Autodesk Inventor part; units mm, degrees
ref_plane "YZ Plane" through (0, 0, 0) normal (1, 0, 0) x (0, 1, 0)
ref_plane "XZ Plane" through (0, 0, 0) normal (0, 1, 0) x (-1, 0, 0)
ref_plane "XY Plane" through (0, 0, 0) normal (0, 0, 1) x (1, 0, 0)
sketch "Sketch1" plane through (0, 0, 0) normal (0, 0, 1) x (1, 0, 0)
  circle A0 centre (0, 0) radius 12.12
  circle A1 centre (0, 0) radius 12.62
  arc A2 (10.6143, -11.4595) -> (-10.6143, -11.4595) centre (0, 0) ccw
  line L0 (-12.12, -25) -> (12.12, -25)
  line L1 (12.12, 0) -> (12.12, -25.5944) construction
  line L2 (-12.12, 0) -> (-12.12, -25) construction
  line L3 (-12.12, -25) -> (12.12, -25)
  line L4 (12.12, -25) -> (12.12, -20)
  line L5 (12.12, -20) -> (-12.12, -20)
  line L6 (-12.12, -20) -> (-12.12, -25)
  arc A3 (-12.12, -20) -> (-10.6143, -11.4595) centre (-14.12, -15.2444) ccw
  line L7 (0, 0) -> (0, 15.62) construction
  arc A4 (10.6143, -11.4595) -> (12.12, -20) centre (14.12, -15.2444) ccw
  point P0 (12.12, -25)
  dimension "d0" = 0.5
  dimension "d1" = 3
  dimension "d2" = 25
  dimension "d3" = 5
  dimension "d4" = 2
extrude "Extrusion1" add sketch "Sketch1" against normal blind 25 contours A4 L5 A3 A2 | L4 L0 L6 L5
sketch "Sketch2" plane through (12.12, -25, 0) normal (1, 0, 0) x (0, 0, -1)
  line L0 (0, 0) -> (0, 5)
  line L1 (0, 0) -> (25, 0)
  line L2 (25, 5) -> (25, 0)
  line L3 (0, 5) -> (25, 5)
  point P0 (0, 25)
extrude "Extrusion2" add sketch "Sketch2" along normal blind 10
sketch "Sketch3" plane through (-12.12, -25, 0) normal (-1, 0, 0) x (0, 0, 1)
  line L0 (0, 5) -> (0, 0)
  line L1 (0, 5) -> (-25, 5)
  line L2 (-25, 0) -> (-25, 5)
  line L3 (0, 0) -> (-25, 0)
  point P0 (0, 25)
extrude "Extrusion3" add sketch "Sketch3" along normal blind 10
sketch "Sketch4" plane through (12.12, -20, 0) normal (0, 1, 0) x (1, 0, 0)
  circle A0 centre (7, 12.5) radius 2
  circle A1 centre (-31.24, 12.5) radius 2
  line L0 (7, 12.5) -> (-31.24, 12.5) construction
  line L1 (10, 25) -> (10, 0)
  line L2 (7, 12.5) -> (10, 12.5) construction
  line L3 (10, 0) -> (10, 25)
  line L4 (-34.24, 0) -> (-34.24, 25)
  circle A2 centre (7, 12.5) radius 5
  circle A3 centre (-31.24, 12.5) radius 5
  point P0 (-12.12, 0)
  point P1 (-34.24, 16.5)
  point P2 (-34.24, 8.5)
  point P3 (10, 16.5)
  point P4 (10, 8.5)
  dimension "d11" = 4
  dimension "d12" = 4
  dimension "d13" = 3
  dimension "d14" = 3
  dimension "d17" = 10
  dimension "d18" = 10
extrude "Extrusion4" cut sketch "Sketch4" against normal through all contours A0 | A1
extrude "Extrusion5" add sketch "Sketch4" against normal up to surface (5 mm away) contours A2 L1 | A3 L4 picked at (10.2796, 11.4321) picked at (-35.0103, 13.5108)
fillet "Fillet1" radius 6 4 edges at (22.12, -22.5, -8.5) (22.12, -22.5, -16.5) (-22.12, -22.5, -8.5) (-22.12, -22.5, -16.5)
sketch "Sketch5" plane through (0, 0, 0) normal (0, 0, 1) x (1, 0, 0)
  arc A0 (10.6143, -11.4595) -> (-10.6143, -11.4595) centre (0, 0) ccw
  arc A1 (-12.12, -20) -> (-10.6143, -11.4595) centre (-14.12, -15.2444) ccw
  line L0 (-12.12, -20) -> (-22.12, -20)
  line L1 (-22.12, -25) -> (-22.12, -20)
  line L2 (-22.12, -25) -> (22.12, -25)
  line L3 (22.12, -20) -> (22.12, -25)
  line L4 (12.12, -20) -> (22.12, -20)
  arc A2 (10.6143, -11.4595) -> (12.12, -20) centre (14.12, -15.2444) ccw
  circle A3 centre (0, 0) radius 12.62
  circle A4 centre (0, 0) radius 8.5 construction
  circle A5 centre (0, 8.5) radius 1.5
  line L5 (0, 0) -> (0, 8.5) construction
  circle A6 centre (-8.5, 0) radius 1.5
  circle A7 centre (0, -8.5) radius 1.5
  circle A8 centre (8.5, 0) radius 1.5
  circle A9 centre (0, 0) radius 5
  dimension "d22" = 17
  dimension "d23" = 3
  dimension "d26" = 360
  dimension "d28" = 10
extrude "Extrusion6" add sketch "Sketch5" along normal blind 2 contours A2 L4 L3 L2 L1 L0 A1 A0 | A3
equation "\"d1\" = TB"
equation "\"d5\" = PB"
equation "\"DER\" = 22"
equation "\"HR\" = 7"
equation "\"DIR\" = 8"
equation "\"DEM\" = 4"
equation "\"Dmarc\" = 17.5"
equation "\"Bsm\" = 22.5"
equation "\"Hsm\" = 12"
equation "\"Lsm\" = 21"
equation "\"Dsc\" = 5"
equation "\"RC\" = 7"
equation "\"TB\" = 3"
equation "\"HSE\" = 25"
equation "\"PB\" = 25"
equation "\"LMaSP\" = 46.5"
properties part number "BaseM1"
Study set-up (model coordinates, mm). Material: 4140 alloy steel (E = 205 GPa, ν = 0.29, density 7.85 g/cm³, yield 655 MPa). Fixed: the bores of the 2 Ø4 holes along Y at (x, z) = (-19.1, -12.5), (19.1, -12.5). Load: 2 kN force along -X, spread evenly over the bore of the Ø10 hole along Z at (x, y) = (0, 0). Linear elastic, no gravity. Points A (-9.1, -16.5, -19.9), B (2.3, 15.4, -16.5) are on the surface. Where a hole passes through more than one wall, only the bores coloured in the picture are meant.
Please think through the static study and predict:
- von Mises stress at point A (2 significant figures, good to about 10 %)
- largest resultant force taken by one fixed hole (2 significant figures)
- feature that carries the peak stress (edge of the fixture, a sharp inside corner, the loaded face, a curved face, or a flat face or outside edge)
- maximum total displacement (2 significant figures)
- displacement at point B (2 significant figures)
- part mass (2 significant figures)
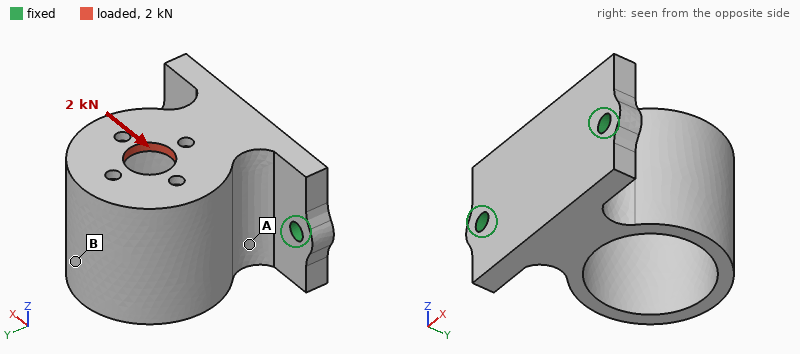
39 MPa
1.9 kN
a curved face
49 µm
49 µm
130 g
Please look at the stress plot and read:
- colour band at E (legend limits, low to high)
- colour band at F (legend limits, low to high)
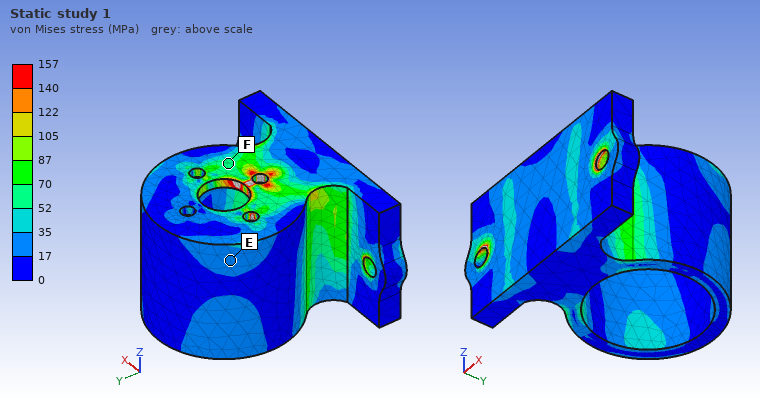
17 to 35 MPa
52 to 70 MPa
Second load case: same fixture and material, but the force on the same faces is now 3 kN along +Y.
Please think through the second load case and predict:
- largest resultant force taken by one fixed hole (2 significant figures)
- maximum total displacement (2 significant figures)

1.6 kN
0.12 mm
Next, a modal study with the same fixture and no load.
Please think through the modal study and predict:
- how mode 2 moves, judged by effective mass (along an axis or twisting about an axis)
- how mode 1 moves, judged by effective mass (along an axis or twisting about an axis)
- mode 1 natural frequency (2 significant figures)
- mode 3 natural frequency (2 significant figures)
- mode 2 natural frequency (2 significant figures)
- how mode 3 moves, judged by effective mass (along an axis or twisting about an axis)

along X
along Z
2800 Hz
8300 Hz
4200 Hz
along Y
